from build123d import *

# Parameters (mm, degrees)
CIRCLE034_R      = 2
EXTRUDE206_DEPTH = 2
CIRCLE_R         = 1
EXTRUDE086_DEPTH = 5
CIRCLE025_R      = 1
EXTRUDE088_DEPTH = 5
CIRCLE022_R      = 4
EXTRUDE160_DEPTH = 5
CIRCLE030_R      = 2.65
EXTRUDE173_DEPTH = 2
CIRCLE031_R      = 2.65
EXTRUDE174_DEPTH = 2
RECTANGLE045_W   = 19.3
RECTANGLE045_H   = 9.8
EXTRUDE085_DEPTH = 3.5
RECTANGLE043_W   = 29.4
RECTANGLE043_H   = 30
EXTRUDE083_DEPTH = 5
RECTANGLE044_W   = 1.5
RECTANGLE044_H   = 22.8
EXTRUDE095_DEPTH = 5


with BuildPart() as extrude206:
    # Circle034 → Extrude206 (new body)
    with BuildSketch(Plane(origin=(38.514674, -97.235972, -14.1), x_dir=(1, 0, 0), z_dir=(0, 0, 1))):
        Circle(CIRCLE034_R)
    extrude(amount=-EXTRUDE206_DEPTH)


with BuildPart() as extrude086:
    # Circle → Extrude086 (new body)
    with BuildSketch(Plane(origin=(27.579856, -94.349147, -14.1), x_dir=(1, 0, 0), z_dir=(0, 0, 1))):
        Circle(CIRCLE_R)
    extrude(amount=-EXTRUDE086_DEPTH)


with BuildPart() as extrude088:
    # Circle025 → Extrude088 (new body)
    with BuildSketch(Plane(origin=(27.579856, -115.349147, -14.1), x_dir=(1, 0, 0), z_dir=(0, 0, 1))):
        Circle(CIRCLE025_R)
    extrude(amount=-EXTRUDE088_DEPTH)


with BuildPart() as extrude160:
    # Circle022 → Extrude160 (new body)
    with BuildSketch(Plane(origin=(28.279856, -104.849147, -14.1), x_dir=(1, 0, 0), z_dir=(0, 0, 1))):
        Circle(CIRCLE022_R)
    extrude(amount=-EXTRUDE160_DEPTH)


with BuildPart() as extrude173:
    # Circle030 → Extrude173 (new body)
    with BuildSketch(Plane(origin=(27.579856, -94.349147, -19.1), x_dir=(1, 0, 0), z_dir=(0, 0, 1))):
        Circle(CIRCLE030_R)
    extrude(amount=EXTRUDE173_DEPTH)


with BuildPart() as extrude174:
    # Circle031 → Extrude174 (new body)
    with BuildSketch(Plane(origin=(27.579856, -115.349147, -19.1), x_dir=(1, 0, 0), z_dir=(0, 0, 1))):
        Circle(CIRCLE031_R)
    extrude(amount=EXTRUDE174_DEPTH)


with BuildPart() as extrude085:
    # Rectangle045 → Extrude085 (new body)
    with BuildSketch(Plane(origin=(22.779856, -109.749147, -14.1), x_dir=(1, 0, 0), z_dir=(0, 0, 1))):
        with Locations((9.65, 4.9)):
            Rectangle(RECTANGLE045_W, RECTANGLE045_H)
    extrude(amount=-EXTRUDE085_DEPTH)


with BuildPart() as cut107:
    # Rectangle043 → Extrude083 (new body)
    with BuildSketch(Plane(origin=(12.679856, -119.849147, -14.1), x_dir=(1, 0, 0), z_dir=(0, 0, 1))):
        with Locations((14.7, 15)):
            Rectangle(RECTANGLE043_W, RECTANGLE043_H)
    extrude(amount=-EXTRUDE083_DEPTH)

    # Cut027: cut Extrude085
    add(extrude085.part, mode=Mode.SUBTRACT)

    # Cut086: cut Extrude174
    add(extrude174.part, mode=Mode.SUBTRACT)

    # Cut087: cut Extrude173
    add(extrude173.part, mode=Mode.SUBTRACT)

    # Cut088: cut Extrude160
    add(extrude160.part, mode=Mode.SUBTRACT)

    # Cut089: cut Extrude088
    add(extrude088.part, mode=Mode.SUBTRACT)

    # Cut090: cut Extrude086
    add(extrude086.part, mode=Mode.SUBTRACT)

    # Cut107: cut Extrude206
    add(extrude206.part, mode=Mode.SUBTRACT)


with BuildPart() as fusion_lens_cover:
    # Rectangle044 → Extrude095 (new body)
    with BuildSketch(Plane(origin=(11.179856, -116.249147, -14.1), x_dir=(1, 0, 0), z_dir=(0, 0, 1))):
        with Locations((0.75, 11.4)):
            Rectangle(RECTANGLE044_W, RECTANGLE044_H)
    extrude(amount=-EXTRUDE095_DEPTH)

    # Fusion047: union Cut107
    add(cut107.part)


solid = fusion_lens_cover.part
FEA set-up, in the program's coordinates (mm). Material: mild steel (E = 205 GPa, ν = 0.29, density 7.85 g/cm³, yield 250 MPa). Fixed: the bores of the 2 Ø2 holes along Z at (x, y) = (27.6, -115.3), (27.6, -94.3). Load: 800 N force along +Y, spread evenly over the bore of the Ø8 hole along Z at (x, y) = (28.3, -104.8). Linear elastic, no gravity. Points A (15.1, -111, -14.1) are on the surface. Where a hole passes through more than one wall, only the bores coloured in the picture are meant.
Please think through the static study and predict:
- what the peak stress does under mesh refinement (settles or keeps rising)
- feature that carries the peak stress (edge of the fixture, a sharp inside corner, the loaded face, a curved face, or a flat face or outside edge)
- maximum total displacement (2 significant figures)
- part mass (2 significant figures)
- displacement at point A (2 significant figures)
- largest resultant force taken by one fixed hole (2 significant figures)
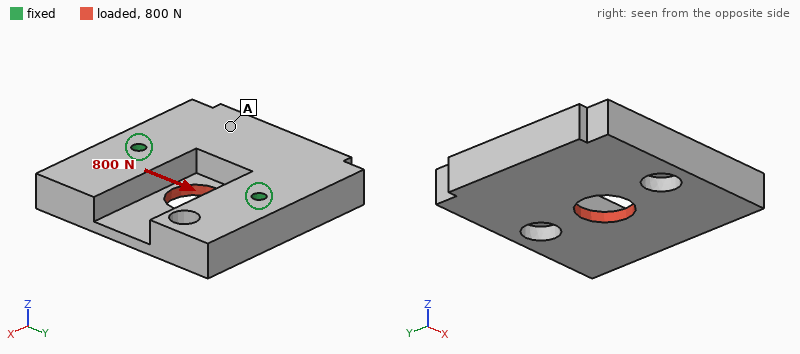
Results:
keeps rising
edge of the fixture
2.0 µm
29 g
0.44 µm
410 N
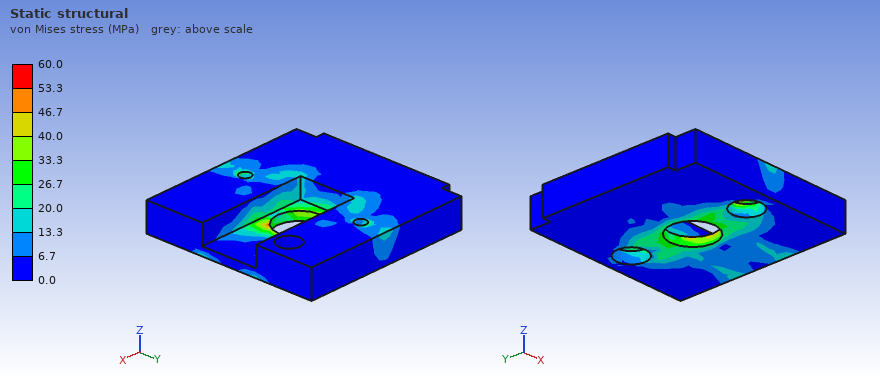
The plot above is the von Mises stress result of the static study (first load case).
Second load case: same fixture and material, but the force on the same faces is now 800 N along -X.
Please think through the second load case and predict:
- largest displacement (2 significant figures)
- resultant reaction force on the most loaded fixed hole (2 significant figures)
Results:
7.7 µm
400 N
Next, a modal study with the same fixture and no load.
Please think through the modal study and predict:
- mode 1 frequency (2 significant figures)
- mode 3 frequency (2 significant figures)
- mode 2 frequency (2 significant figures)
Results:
7100 Hz
14 kHz
14 kHz
